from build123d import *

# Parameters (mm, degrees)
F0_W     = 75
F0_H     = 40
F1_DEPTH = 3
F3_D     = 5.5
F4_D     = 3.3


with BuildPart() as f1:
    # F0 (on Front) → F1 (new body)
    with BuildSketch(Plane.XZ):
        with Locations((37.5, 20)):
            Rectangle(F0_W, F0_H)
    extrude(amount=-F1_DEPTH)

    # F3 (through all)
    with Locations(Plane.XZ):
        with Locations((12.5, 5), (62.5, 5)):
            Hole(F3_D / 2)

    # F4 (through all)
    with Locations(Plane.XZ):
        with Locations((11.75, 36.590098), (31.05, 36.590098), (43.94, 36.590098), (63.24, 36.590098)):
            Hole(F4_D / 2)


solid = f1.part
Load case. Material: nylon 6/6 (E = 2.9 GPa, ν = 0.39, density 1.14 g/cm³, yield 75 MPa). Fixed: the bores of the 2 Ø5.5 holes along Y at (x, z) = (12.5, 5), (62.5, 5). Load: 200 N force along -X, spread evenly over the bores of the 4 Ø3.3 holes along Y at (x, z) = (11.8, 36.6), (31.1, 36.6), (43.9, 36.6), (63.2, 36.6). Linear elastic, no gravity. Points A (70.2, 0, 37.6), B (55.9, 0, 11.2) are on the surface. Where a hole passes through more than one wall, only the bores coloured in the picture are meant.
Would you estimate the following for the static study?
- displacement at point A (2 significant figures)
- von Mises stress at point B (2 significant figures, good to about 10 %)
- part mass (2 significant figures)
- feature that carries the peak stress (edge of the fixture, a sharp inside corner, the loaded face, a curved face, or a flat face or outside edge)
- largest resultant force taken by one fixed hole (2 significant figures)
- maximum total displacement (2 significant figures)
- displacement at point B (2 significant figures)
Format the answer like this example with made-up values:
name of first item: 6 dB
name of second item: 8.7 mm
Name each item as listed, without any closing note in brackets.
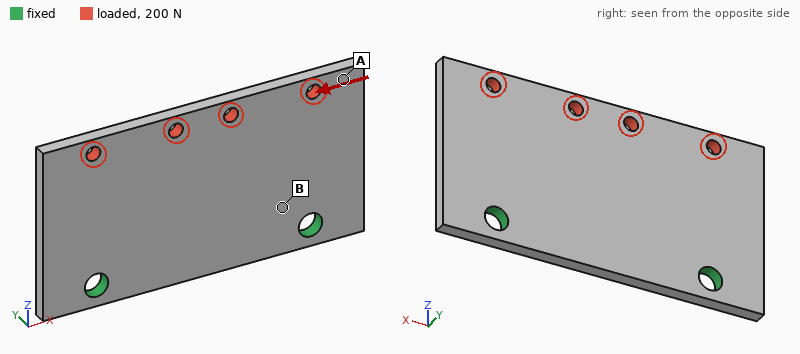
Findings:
displacement at point A: 58 µm
von Mises stress at point B: 3.0 MPa
part mass: 10.0 g
feature that carries the peak stress: edge of the fixture
largest resultant force taken by one fixed hole: 150 N
maximum total displacement: 64 µm
displacement at point B: 9.9 µm
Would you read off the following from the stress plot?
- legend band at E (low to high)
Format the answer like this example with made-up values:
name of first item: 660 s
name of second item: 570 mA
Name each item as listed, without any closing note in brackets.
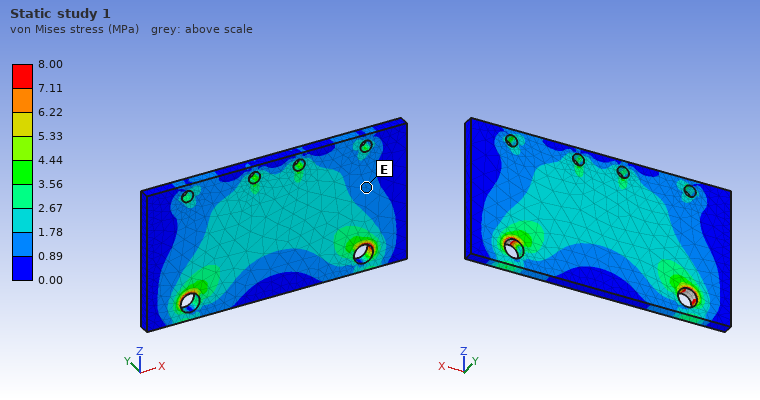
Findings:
legend band at E: 0.89 to 1.78 MPa
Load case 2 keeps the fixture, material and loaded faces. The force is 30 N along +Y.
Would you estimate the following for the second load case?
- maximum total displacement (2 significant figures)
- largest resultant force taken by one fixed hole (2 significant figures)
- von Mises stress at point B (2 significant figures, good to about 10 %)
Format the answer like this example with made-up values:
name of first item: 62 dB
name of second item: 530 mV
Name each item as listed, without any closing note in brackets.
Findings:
maximum total displacement: 0.98 mm
largest resultant force taken by one fixed hole: 15 N
von Mises stress at point B: 7.3 MPa
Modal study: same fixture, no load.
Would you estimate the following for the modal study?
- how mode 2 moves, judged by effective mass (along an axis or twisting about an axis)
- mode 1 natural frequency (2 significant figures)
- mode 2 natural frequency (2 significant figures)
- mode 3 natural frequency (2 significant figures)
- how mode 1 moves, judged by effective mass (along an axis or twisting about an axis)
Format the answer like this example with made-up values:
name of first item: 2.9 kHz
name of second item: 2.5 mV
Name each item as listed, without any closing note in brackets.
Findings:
how mode 2 moves, judged by effective mass: twisting about Z
mode 1 natural frequency: 580 Hz
mode 2 natural frequency: 950 Hz
mode 3 natural frequency: 1500 Hz
how mode 1 moves, judged by effective mass: along Y
